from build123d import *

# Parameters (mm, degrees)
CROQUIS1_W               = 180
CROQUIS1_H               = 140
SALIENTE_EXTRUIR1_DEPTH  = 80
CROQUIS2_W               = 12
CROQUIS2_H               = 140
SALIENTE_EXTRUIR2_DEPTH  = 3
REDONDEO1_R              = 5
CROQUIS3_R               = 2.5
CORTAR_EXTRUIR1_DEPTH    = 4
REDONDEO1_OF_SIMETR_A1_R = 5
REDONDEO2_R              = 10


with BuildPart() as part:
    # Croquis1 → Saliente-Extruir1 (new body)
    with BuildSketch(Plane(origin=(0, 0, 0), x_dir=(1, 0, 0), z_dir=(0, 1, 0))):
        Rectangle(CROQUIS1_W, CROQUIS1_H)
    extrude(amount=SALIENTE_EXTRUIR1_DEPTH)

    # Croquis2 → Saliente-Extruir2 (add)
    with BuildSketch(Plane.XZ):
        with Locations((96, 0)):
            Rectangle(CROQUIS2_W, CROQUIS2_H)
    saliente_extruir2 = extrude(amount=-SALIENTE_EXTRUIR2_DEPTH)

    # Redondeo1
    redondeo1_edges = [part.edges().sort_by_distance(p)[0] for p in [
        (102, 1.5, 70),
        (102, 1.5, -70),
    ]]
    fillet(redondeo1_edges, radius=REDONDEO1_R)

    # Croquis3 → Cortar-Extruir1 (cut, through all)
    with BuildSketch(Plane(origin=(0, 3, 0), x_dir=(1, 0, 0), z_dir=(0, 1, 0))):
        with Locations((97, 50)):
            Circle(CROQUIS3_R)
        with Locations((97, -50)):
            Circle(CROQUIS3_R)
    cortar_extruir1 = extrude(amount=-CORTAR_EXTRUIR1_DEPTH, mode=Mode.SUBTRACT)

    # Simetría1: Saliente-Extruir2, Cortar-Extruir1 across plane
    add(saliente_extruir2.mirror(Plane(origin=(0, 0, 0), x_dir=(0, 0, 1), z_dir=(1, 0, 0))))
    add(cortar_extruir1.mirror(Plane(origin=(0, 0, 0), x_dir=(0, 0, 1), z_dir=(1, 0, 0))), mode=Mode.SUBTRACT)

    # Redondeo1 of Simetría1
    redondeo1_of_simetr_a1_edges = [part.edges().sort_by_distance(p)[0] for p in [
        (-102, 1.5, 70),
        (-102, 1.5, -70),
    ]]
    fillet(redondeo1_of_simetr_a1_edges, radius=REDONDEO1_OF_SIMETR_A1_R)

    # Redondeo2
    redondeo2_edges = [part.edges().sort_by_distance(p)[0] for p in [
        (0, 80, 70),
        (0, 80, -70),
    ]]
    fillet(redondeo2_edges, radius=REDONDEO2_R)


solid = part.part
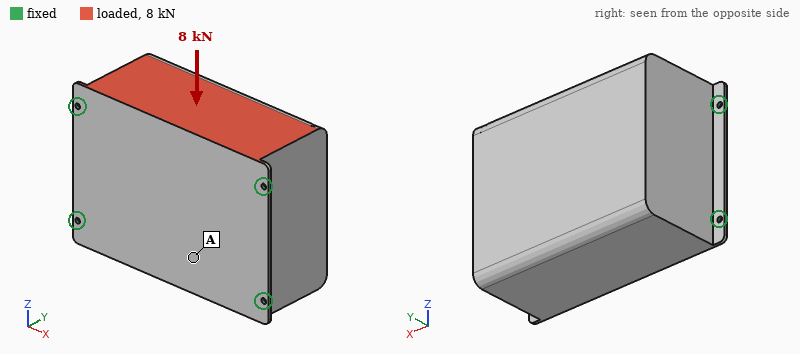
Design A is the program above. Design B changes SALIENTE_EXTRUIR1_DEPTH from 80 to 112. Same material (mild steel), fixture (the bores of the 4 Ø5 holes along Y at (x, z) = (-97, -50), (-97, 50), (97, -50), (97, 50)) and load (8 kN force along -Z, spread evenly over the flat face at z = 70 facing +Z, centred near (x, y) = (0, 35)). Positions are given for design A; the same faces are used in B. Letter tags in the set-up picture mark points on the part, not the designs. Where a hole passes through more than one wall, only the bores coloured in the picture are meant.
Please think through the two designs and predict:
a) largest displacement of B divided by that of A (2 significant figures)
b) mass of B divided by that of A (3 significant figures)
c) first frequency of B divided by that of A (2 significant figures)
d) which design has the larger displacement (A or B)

1.8
1.40
0.68
B
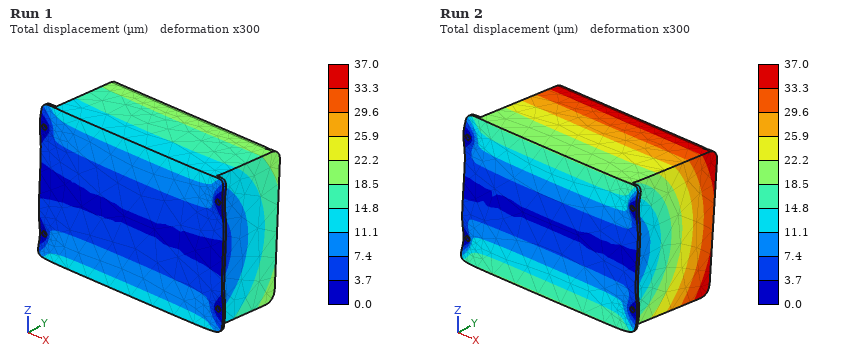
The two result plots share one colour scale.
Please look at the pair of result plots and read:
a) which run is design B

Run 2
